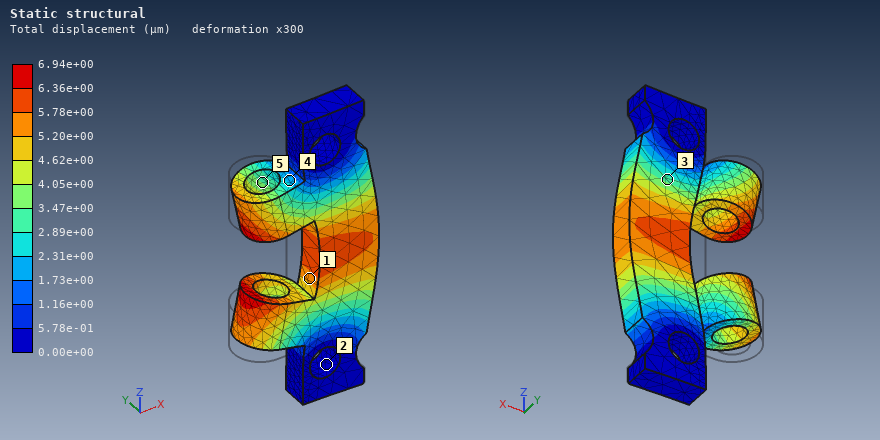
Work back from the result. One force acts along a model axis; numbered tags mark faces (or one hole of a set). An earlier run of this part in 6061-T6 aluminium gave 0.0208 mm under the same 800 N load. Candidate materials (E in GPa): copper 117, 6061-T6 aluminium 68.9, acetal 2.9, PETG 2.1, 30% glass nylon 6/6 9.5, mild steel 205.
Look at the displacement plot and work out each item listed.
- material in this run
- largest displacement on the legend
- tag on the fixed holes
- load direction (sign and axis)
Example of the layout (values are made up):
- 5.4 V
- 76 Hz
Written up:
- mild steel
- 6.94e+00 µm
- 2
- +X
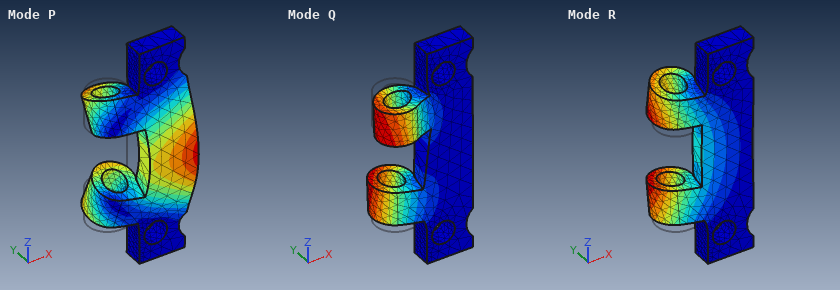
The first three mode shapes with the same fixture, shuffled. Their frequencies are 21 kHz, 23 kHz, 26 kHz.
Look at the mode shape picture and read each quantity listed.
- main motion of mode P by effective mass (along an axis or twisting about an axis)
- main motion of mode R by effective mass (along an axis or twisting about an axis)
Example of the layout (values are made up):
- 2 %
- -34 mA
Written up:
- along Y
- along Y
